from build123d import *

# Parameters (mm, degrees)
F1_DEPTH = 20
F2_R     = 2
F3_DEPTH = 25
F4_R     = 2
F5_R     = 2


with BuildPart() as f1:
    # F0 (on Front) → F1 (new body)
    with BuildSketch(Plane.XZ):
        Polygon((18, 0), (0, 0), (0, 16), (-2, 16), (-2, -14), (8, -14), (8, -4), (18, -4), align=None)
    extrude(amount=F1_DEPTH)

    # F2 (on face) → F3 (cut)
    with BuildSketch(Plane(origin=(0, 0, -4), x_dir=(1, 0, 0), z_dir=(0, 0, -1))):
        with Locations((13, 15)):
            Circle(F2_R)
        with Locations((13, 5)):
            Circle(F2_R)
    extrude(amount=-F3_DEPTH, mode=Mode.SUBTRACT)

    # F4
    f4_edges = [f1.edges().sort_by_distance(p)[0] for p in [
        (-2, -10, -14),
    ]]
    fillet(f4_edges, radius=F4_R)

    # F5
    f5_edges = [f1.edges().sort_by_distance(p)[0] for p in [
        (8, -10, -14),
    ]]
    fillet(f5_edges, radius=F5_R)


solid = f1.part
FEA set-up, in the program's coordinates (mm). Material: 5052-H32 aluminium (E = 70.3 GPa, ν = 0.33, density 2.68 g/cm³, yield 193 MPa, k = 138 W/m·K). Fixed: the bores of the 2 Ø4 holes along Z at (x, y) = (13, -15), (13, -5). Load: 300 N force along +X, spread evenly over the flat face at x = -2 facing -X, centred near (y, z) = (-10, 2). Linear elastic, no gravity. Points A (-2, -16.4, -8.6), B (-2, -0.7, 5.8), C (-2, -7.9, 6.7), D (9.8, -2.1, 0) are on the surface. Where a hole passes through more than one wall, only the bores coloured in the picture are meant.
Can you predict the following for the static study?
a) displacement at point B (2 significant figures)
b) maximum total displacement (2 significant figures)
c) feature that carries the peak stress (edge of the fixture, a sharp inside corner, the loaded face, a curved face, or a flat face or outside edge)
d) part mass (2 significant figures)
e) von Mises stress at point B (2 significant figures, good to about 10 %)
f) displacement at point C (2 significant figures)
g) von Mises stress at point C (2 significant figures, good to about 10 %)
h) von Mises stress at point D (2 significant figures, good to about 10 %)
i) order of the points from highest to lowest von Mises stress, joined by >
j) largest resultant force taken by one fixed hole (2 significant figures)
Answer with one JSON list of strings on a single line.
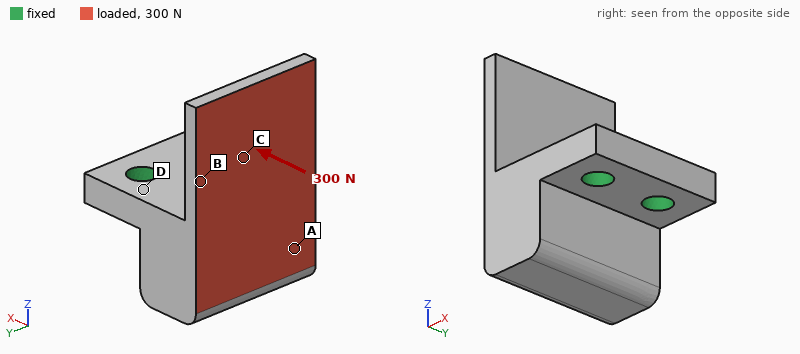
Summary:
["0.040 mm", "0.14 mm", "the loaded face", "11 g", "43 MPa", "0.049 mm", "32 MPa", "21 MPa", "B > C > D > A", "150 N"]
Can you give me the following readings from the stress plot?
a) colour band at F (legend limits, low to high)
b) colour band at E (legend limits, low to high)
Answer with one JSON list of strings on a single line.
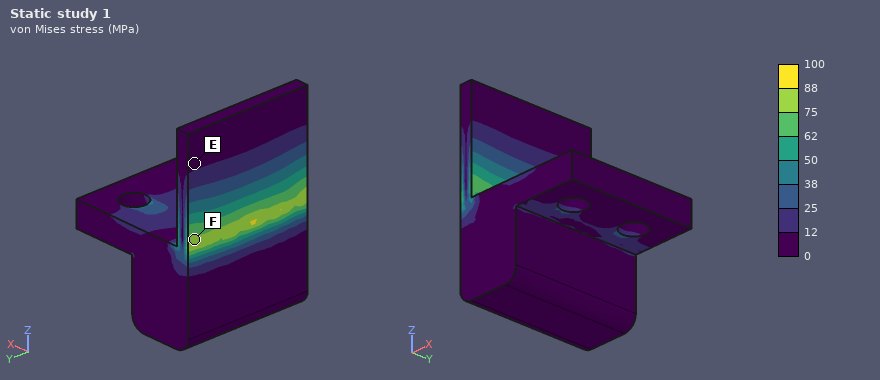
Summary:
["75 to 88 MPa", "0 to 12 MPa"]
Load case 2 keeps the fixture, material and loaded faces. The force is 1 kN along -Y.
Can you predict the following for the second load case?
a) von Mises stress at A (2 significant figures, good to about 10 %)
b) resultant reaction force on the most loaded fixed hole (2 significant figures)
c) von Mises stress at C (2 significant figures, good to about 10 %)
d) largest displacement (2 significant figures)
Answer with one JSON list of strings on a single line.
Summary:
["14 MPa", "1.2 kN", "34 MPa", "58 µm"]
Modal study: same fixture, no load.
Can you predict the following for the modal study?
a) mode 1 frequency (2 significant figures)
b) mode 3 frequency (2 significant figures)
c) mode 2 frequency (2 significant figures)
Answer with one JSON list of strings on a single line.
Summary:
["4700 Hz", "12 kHz", "7600 Hz"]
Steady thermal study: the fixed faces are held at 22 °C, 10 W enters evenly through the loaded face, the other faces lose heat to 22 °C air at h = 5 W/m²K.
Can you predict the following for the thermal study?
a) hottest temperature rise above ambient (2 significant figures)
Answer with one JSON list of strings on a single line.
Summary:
["18 K"]
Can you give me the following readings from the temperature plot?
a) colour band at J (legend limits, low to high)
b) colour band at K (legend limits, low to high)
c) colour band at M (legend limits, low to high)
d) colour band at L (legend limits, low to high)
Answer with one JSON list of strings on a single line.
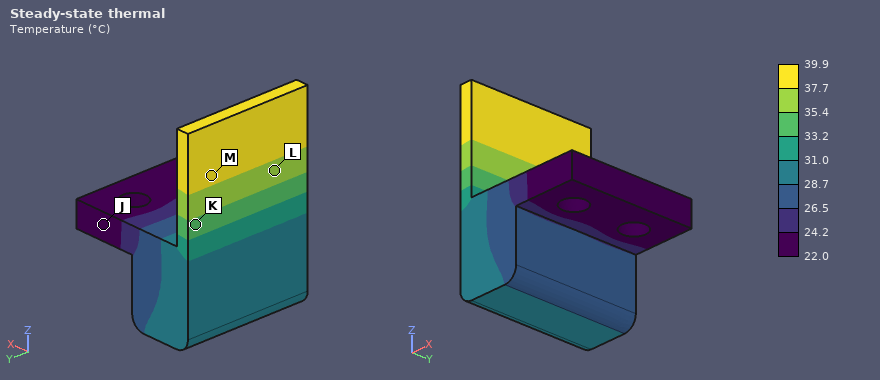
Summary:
["22.0 to 24.2 °C", "33.2 to 35.4 °C", "37.7 to 39.9 °C", "35.4 to 37.7 °C"]
